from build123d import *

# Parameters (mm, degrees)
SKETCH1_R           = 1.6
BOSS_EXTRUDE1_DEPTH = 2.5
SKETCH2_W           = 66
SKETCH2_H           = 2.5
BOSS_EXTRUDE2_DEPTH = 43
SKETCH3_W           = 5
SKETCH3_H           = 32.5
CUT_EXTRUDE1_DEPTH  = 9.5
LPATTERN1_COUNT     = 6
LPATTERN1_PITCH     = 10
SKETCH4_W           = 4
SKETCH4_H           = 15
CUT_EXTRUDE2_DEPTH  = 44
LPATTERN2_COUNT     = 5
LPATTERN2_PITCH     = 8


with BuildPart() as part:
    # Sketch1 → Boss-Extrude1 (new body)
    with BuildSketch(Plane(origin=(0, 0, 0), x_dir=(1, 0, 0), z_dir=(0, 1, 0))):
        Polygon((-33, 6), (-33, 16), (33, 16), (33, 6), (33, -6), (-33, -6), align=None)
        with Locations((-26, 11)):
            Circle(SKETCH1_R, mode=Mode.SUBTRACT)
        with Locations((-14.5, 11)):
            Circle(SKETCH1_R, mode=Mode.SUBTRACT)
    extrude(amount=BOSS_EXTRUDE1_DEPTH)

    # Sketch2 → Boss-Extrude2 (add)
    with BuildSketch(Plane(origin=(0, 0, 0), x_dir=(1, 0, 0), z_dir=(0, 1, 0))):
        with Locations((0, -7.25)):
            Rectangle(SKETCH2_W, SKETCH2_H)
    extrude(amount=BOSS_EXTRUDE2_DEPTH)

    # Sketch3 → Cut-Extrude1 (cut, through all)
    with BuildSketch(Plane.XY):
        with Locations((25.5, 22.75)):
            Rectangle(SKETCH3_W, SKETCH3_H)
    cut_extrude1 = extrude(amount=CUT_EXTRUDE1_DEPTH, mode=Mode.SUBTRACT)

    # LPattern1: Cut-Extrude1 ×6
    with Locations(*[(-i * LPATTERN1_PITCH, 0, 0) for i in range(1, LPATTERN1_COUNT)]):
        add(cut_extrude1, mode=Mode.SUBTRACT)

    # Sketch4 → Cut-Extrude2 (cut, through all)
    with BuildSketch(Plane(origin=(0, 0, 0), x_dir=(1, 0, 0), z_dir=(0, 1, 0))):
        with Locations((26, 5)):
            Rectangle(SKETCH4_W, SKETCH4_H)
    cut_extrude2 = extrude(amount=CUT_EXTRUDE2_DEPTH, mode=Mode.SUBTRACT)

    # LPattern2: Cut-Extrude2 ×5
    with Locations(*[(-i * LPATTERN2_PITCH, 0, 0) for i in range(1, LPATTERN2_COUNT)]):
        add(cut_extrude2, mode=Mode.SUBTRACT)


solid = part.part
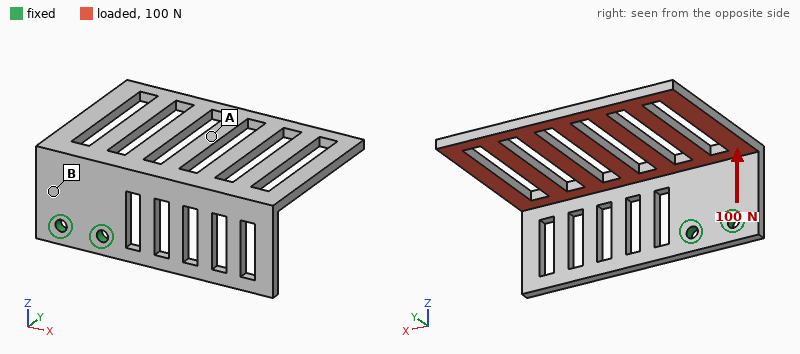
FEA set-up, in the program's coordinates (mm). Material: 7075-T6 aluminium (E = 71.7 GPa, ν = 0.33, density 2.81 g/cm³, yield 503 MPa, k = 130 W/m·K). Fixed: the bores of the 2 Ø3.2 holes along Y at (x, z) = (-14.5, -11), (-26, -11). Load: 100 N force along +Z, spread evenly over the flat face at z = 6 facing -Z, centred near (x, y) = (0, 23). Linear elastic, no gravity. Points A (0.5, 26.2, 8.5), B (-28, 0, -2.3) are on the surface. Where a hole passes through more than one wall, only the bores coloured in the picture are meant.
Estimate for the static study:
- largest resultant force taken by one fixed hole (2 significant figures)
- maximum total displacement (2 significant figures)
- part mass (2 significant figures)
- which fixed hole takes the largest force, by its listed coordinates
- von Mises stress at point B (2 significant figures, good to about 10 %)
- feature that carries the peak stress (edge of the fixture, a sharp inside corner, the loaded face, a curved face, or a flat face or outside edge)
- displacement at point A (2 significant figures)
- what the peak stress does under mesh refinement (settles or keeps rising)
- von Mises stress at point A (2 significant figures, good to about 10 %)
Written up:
190 N
0.95 mm
21 g
(-14.5, -11)
56 MPa
edge of the fixture
0.49 mm
keeps rising
13 MPa
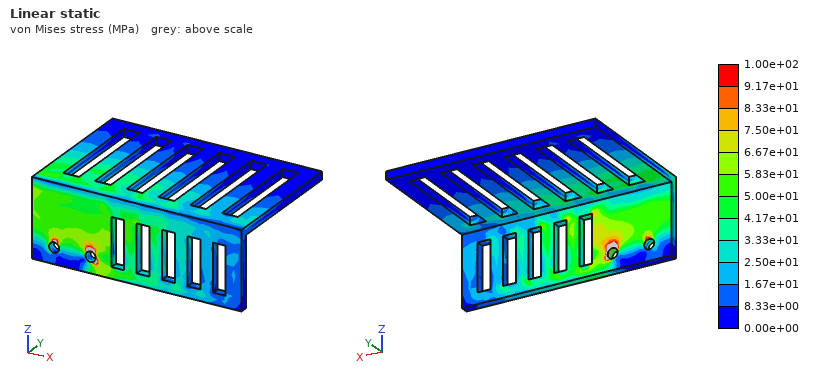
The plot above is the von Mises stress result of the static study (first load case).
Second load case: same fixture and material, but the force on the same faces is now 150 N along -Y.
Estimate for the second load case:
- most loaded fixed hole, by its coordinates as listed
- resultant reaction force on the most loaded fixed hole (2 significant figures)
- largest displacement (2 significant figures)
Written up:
(-14.5, -11)
250 N
0.76 mm
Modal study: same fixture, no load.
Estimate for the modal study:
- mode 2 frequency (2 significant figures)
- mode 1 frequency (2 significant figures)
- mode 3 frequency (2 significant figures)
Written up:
730 Hz
530 Hz
1400 Hz
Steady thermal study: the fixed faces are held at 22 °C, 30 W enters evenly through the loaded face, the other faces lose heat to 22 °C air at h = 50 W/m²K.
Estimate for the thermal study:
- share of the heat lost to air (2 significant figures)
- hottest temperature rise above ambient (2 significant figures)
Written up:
50 %
80 K
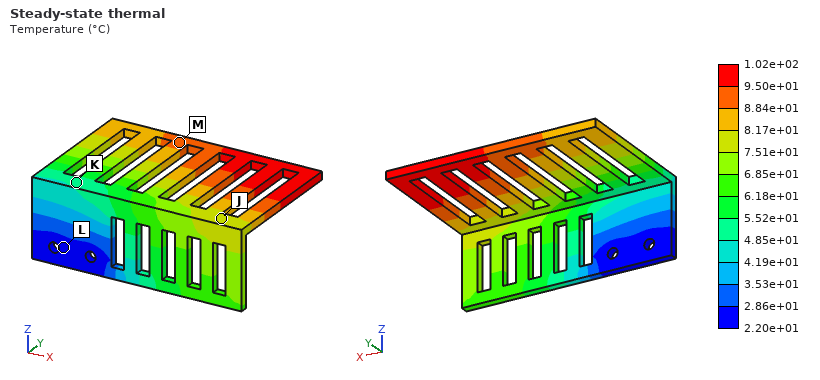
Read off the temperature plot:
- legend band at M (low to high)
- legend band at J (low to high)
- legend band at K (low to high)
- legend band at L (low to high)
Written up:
8.84e+01 to 9.50e+01 °C
7.51e+01 to 8.17e+01 °C
4.85e+01 to 5.52e+01 °C
2.20e+01 to 2.86e+01 °C
